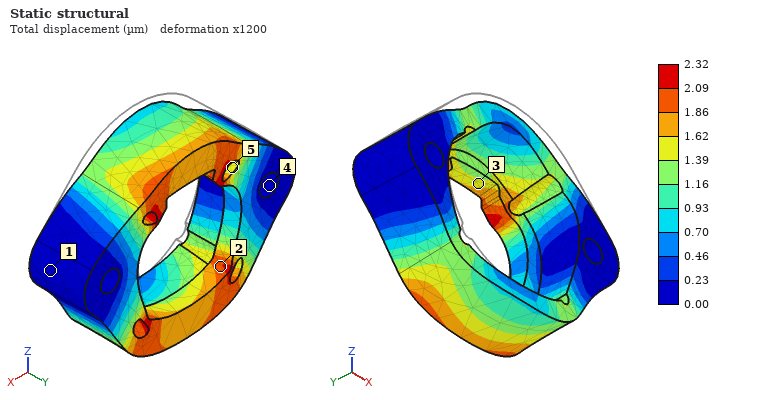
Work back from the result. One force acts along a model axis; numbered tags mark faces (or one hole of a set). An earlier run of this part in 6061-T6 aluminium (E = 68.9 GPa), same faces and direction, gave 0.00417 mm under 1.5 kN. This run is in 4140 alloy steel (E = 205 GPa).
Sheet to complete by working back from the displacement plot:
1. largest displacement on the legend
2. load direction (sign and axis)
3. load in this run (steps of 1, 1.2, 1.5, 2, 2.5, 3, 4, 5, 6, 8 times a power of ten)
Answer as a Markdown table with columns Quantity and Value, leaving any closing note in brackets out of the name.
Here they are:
| Quantity | Value |
|---|---|
| largest displacement on the legend | 2.32 µm |
| load direction | -Z |
| load in this run | 2.5 kN |
